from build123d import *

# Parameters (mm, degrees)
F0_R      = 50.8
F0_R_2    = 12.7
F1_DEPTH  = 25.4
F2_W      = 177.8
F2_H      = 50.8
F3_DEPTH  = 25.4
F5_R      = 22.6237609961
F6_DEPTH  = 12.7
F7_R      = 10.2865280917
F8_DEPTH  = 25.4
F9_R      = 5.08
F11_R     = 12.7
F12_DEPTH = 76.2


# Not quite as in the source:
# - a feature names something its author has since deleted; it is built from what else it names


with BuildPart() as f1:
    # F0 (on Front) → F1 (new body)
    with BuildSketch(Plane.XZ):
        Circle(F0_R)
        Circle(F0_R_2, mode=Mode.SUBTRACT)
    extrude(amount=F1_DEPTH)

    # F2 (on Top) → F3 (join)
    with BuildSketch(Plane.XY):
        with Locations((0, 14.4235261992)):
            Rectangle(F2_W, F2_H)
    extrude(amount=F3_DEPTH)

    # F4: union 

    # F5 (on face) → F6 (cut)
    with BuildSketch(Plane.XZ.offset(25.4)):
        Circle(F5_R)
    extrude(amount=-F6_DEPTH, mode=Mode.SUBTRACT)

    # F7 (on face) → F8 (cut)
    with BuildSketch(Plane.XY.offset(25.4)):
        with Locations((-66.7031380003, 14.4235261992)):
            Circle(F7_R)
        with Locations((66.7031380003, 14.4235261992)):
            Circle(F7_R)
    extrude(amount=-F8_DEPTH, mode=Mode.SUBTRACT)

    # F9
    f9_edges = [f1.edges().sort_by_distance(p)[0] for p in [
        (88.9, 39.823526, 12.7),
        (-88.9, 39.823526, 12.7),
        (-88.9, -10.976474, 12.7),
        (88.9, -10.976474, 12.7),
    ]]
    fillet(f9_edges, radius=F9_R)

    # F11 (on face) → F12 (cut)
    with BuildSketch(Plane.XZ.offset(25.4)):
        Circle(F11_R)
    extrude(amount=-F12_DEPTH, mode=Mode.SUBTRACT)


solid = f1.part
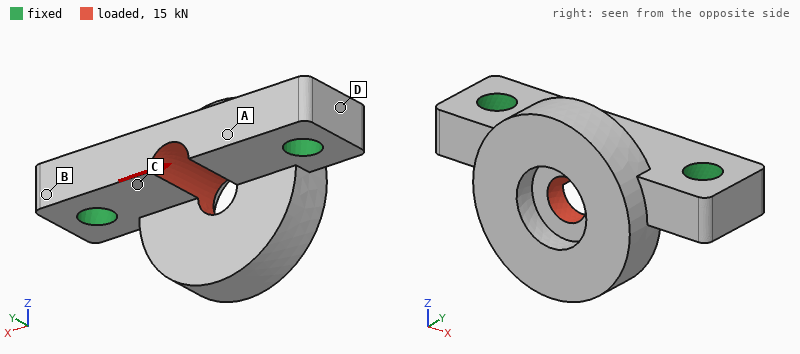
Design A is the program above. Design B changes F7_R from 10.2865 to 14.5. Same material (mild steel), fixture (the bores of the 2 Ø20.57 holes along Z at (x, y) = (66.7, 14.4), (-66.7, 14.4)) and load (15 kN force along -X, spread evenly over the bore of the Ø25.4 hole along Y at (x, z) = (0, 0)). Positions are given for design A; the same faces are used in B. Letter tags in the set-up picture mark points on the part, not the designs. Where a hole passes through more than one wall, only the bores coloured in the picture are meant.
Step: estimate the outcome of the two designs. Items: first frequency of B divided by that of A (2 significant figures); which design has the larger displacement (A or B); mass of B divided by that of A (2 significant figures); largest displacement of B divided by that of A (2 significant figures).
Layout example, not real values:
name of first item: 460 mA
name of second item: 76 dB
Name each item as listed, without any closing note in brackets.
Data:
first frequency of B divided by that of A: 1.1
which design has the larger displacement: A
mass of B divided by that of A: 0.95
largest displacement of B divided by that of A: 0.90
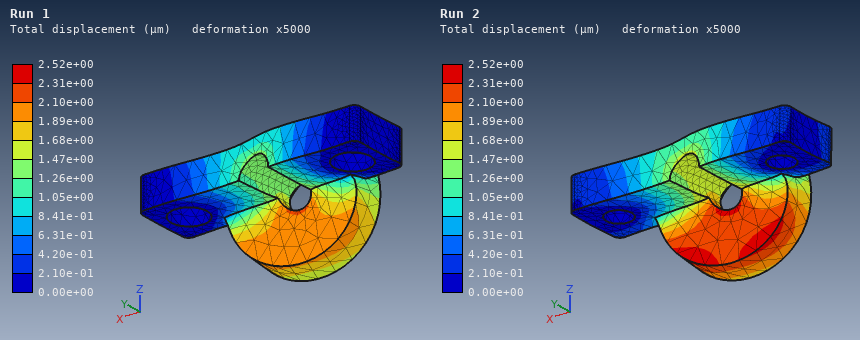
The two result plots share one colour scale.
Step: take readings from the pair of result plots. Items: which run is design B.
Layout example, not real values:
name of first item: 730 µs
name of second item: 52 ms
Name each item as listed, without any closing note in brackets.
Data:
which run is design B: Run 1
